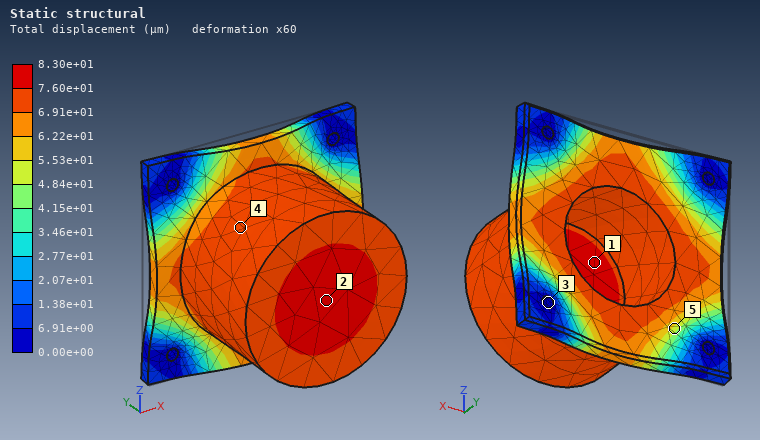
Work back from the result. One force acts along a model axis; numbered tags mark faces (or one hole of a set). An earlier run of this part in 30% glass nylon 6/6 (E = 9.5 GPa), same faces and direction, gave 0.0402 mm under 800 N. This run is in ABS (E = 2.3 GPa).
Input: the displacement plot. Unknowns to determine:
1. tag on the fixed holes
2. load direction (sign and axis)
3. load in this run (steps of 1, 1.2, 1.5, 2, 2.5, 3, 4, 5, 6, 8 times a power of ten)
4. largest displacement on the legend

3
-Y
400 N
8.30e+01 µm
